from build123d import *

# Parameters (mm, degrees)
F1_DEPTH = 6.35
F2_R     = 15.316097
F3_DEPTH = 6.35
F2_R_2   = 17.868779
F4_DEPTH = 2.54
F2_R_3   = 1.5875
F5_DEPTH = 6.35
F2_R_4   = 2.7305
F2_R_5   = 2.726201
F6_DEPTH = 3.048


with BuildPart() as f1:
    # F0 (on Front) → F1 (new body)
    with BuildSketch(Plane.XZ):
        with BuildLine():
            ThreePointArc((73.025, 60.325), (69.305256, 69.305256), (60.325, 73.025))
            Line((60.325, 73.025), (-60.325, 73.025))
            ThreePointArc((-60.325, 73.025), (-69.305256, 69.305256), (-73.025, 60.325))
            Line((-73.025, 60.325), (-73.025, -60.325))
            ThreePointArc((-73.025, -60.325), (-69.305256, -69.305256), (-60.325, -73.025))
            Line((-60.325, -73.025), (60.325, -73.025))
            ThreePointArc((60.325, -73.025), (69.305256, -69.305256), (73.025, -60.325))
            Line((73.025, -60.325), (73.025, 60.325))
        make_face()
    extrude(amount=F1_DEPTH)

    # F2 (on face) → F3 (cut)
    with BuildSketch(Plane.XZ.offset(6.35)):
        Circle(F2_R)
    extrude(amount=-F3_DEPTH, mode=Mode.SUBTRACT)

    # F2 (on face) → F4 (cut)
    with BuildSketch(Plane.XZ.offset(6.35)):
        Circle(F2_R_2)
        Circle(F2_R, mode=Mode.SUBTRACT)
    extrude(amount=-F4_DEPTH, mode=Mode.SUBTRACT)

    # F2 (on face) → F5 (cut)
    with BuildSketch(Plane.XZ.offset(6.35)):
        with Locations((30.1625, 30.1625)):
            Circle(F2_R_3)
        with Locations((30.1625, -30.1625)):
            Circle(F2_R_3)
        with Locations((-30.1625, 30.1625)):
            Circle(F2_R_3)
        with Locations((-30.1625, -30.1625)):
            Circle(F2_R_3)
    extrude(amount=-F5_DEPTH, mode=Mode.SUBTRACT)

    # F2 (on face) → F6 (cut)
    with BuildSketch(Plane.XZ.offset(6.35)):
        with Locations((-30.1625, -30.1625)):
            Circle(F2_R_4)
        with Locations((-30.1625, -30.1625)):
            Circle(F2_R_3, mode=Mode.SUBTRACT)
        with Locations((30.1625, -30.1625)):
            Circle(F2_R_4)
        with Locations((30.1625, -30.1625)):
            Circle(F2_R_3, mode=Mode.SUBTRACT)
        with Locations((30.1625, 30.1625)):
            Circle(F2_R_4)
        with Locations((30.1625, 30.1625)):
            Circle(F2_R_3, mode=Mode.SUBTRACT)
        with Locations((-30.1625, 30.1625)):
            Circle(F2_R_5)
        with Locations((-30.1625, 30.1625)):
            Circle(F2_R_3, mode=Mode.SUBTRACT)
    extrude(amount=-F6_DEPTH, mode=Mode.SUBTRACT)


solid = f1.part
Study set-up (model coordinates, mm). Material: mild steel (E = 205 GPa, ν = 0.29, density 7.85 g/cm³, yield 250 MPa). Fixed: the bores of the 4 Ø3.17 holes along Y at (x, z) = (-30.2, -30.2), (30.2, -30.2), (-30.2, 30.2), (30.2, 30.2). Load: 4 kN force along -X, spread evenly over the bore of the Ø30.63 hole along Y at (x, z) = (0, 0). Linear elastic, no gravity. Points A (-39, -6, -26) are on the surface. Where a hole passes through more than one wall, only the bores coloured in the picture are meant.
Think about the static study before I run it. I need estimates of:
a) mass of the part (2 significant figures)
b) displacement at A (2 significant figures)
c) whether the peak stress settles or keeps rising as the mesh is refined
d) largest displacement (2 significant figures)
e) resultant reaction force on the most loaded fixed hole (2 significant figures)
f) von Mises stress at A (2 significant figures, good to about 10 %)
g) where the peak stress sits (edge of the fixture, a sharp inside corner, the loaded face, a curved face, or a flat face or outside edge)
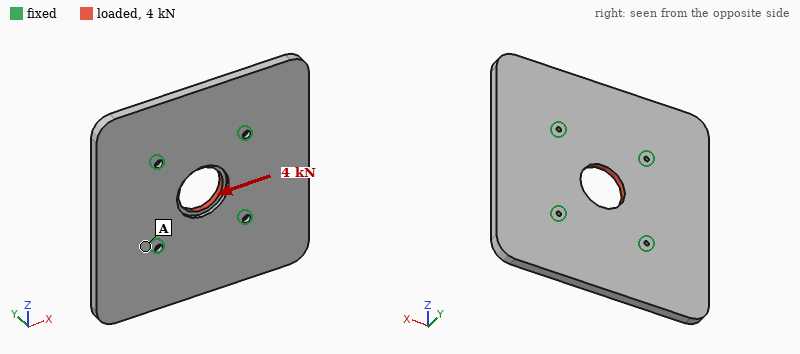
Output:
1.0 kg
0.89 µm
keeps rising
2.2 µm
1.0 kN
4.1 MPa
edge of the fixture
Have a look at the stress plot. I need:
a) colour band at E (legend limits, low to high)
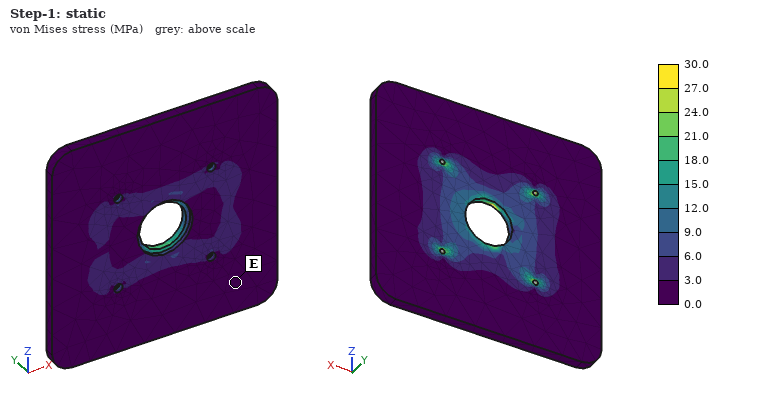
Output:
0.0 to 3.0 MPa
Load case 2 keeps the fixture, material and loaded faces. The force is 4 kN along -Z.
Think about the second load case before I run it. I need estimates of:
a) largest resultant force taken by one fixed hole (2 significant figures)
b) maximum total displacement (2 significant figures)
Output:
1.0 kN
2.2 µm
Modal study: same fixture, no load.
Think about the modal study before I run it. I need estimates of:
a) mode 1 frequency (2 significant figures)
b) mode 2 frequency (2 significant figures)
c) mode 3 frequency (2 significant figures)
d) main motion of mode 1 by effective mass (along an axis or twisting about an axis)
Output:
1600 Hz
1800 Hz
1800 Hz
along Y
